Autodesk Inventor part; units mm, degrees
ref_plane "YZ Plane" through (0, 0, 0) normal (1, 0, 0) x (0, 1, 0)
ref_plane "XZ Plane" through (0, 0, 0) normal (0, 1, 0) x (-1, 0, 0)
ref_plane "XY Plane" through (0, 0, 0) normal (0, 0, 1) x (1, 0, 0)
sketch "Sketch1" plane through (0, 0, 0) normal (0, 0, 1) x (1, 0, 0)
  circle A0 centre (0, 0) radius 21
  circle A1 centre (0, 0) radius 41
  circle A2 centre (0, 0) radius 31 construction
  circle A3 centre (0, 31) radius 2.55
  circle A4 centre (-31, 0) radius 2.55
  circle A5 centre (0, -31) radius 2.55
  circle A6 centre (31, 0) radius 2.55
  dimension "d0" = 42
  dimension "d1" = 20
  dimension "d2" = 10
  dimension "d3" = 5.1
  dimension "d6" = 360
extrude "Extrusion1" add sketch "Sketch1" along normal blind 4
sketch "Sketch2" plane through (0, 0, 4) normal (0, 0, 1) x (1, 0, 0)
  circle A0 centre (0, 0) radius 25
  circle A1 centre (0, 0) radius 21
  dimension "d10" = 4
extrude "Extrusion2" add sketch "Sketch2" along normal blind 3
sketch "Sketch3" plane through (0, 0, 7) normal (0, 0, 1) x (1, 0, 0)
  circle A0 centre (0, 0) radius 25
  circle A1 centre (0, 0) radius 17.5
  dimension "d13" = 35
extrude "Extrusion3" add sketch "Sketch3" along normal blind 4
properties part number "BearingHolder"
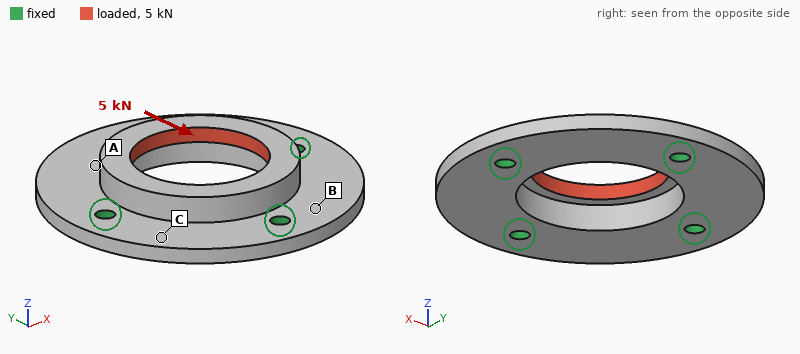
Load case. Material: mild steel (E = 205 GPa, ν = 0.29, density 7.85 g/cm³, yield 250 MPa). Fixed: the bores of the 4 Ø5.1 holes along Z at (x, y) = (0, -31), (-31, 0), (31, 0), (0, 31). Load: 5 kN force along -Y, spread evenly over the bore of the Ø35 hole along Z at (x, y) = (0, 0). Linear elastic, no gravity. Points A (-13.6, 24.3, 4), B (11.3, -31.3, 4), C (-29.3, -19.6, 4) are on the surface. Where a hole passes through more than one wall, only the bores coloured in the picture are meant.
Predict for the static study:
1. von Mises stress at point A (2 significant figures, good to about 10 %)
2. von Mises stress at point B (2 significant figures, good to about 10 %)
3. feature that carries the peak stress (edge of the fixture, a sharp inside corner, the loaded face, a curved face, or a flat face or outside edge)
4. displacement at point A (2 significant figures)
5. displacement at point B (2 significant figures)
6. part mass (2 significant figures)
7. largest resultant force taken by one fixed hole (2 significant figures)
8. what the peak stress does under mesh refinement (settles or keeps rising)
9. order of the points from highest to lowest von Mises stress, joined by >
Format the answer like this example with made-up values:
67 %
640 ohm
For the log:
17 MPa
9.4 MPa
edge of the fixture
2.2 µm
1.8 µm
160 g
1.4 kN
keeps rising
A > B > C
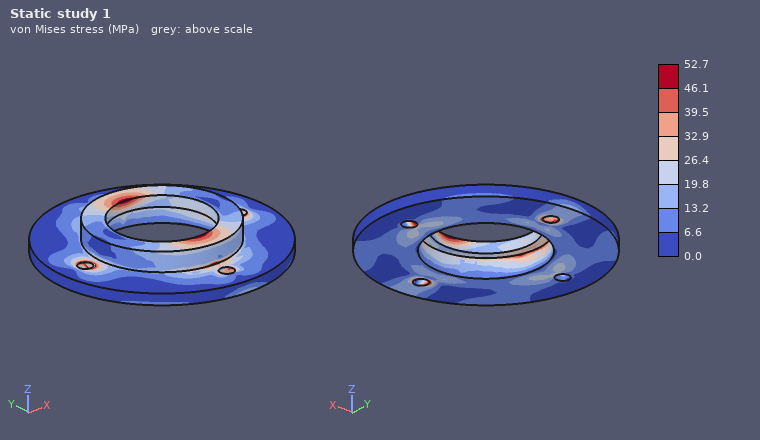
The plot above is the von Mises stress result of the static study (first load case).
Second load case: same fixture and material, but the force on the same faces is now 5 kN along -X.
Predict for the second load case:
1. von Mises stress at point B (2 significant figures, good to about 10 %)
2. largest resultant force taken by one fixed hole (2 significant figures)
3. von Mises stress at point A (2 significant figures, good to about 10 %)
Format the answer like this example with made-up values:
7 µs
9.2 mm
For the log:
8.8 MPa
1.4 kN
8.6 MPa
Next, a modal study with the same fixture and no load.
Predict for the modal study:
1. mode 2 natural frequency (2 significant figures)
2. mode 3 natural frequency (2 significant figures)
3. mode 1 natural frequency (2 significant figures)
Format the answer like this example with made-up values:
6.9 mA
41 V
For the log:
9100 Hz
9100 Hz
8000 Hz
